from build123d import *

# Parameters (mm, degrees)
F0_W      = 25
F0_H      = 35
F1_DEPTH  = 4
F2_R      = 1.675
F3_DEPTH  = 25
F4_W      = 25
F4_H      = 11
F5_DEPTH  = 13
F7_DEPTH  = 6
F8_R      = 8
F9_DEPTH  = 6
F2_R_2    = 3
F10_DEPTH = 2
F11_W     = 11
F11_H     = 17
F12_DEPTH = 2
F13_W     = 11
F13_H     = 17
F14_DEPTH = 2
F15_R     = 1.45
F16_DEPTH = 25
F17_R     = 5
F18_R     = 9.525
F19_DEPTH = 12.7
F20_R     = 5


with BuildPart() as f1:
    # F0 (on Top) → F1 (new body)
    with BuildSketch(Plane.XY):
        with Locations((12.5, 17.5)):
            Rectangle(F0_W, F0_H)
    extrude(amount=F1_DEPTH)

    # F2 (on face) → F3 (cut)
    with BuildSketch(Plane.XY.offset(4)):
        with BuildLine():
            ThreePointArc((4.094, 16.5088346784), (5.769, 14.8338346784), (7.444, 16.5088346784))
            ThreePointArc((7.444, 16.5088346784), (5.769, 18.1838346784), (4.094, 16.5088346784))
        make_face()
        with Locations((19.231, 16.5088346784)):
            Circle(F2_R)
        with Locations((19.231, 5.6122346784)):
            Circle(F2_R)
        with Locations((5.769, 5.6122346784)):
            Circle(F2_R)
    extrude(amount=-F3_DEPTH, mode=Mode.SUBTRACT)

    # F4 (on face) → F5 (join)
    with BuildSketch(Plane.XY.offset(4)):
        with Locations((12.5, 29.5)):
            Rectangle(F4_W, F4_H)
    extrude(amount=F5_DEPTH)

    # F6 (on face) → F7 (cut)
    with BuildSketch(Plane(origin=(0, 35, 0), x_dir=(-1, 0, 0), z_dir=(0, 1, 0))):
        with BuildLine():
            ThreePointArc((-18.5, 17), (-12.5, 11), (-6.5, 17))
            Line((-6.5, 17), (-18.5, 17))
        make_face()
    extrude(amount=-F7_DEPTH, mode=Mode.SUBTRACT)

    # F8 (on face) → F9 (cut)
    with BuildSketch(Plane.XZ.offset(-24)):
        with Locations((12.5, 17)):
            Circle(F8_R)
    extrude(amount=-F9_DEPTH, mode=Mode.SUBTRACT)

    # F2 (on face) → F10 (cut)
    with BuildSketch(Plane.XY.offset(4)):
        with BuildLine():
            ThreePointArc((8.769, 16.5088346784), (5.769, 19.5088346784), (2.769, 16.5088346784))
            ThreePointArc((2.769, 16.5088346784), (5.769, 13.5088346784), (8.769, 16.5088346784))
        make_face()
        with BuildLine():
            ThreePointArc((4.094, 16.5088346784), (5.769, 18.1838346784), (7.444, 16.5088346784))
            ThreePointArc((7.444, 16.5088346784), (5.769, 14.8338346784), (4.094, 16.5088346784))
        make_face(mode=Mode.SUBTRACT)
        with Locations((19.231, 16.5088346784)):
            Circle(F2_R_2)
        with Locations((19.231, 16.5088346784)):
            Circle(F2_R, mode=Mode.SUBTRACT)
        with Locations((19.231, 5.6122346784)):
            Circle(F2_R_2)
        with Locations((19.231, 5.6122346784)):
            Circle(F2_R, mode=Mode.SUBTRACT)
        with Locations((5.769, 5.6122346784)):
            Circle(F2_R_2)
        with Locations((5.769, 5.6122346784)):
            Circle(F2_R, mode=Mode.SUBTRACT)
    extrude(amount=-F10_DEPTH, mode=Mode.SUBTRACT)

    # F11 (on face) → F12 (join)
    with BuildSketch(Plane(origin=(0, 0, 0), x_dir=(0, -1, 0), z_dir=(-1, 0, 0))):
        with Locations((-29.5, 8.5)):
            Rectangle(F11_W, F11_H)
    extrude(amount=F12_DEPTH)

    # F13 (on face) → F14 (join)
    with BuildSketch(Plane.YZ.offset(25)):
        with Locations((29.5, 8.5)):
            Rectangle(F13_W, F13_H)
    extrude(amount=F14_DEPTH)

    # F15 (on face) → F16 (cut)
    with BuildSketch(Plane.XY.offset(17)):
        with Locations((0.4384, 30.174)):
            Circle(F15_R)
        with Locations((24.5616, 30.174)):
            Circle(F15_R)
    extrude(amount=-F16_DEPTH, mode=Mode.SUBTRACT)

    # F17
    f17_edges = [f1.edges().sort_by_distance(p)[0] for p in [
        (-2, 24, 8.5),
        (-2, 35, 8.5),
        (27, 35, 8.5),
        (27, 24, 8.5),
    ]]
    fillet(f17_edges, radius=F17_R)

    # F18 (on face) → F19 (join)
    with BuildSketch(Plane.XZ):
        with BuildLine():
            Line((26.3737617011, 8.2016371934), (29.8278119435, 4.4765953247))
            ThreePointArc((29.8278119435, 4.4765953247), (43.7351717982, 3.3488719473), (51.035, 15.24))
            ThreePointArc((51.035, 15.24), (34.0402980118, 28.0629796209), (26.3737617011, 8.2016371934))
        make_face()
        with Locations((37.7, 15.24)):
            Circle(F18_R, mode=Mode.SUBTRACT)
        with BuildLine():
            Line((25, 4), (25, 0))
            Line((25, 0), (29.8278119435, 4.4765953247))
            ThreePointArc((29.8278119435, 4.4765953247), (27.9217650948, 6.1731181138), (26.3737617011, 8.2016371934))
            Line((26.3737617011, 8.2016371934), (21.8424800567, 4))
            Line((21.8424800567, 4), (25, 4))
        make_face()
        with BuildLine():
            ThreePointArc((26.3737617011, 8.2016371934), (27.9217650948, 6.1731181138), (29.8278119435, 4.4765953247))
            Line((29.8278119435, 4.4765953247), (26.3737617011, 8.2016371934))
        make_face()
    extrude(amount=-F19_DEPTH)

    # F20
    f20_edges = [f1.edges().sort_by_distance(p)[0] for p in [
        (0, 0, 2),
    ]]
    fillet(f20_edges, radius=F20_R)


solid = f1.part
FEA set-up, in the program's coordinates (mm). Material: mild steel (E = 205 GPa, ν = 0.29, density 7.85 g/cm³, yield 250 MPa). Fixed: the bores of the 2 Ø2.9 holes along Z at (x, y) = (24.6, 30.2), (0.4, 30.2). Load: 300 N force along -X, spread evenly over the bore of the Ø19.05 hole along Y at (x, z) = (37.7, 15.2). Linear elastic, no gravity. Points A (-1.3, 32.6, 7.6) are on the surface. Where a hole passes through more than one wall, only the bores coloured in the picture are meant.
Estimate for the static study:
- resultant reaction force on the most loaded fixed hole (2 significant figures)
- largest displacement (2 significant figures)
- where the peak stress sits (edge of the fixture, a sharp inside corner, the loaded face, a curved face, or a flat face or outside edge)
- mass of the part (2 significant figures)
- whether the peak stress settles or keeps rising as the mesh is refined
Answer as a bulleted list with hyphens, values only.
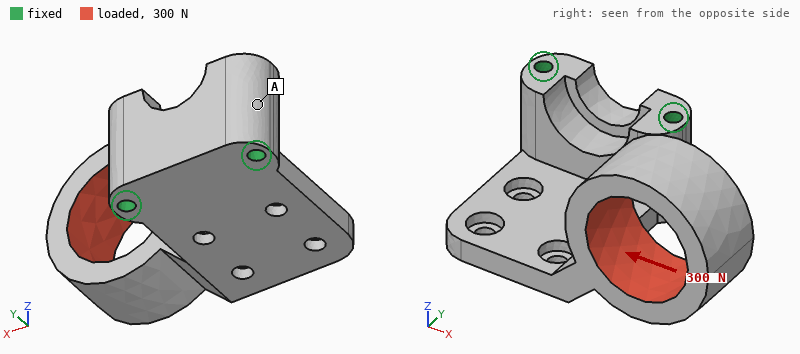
- 370 N
- 0.17 mm
- a sharp inside corner
- 77 g
- keeps rising
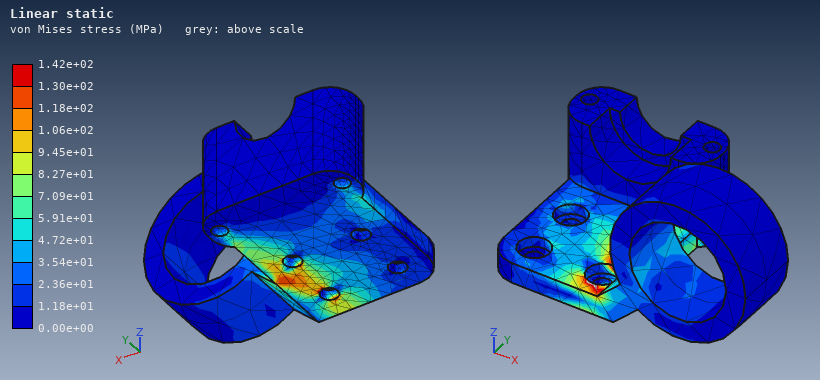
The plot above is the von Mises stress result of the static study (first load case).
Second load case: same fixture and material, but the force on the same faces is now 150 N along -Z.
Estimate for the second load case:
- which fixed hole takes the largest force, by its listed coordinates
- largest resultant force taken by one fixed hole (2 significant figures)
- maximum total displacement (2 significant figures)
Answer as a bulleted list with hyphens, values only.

- (24.6, 30.2)
- 250 N
- 0.14 mm
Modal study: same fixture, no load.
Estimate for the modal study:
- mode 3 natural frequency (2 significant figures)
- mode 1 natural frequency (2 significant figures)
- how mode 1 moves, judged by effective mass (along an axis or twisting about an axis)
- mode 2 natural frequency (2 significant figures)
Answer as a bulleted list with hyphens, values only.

- 4600 Hz
- 1000 Hz
- along Z
- 1700 Hz
